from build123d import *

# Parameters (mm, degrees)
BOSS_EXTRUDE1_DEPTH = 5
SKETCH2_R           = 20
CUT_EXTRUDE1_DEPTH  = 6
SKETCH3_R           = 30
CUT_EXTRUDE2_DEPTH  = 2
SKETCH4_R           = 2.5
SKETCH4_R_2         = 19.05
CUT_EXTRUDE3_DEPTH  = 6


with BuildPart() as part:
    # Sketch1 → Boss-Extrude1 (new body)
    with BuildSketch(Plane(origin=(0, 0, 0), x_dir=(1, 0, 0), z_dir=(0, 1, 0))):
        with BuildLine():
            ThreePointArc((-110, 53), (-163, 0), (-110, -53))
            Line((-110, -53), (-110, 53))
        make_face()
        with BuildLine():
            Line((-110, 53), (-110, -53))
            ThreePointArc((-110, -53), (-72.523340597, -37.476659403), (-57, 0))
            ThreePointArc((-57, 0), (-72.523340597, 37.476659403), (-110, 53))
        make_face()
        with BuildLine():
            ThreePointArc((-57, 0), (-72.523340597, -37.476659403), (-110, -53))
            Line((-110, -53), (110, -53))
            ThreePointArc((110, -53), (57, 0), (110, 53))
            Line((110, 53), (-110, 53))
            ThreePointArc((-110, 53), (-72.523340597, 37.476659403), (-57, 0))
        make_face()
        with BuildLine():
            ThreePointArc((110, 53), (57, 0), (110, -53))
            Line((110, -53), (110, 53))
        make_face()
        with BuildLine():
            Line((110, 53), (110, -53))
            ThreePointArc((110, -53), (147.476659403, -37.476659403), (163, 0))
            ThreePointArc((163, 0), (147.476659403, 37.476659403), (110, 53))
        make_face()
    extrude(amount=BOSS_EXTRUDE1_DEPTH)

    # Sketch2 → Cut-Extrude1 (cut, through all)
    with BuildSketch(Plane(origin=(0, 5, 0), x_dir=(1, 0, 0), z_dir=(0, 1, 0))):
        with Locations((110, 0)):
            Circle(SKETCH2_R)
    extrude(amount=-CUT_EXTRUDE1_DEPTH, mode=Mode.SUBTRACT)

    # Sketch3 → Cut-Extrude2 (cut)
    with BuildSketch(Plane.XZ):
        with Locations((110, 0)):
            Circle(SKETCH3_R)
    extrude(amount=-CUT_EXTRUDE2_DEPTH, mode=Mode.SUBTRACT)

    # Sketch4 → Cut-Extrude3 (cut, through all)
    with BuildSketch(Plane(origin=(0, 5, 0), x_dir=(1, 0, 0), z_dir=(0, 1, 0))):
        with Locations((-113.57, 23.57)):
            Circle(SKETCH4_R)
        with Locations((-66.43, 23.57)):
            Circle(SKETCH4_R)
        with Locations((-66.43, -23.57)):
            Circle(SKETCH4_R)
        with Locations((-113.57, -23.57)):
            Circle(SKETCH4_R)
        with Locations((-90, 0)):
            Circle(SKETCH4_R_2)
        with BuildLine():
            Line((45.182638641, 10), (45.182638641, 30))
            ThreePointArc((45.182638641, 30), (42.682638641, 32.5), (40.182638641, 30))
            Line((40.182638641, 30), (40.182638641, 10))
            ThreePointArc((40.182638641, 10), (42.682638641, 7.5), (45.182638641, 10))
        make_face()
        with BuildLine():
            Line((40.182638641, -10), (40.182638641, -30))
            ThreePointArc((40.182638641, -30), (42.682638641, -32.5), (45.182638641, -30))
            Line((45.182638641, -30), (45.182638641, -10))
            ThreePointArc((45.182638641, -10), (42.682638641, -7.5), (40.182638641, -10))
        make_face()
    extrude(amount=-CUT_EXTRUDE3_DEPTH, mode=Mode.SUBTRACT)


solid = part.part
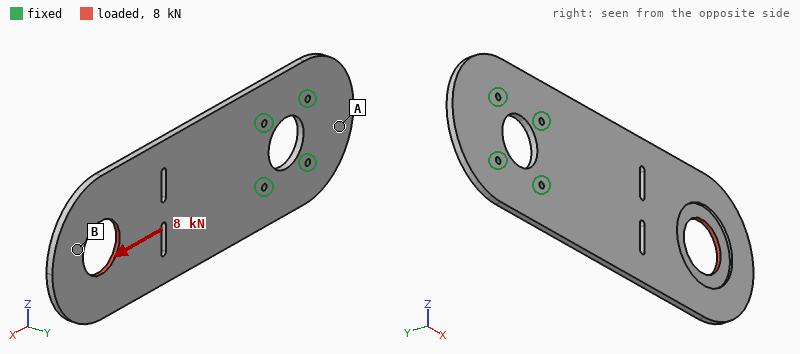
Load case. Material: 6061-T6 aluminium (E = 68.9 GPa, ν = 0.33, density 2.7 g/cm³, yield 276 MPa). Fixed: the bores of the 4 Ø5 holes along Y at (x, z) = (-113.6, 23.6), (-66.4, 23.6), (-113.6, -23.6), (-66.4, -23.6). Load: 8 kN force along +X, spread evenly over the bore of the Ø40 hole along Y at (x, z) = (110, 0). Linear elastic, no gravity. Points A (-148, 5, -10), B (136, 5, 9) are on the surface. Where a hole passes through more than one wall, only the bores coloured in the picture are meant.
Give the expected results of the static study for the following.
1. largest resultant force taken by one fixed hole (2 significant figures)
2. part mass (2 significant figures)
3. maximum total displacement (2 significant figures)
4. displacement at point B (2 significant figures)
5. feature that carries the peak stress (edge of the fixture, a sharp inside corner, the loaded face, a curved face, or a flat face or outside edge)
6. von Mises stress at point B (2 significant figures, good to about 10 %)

3.3 kN
390 g
2.8 mm
2.3 mm
a curved face
17 MPa
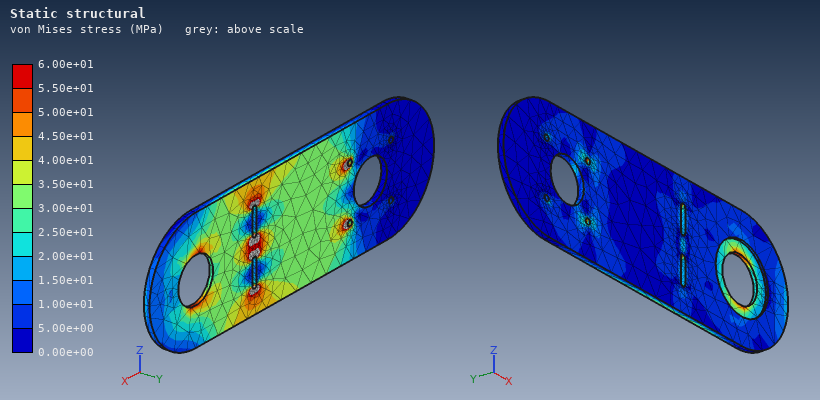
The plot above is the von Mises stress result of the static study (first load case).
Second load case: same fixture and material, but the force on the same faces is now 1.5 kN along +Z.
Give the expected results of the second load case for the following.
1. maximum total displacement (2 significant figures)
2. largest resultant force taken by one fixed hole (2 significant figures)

0.21 mm
3.3 kN
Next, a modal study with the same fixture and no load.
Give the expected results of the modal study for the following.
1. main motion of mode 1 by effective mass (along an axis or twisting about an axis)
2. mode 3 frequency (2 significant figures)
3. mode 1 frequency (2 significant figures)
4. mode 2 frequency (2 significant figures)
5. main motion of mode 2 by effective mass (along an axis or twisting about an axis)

along Y
470 Hz
91 Hz
380 Hz
twisting about X
